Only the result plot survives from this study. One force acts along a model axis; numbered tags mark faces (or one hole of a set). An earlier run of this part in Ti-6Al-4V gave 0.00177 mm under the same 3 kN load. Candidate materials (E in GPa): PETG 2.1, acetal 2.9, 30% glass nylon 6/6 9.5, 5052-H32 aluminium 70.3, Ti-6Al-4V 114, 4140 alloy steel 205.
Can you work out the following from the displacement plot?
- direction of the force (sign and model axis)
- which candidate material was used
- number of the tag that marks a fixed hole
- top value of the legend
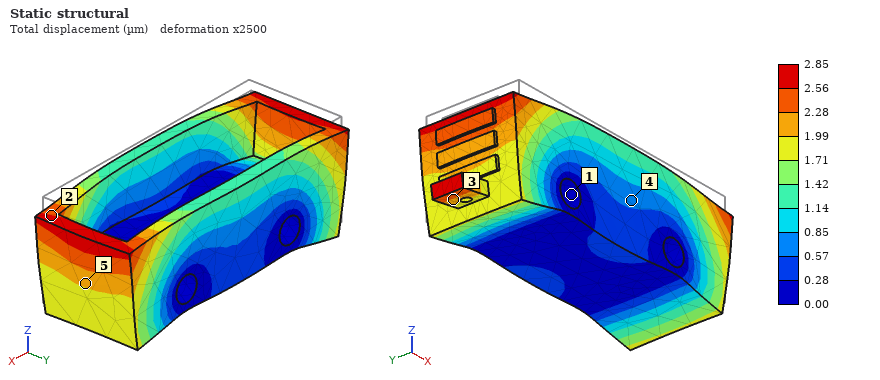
-Z
5052-H32 aluminium
1
2.85 µm
